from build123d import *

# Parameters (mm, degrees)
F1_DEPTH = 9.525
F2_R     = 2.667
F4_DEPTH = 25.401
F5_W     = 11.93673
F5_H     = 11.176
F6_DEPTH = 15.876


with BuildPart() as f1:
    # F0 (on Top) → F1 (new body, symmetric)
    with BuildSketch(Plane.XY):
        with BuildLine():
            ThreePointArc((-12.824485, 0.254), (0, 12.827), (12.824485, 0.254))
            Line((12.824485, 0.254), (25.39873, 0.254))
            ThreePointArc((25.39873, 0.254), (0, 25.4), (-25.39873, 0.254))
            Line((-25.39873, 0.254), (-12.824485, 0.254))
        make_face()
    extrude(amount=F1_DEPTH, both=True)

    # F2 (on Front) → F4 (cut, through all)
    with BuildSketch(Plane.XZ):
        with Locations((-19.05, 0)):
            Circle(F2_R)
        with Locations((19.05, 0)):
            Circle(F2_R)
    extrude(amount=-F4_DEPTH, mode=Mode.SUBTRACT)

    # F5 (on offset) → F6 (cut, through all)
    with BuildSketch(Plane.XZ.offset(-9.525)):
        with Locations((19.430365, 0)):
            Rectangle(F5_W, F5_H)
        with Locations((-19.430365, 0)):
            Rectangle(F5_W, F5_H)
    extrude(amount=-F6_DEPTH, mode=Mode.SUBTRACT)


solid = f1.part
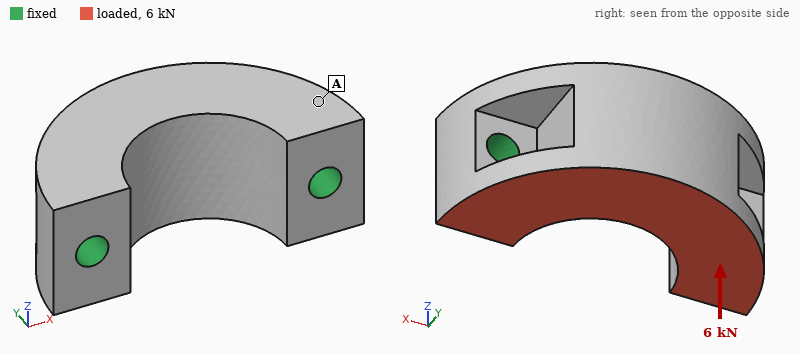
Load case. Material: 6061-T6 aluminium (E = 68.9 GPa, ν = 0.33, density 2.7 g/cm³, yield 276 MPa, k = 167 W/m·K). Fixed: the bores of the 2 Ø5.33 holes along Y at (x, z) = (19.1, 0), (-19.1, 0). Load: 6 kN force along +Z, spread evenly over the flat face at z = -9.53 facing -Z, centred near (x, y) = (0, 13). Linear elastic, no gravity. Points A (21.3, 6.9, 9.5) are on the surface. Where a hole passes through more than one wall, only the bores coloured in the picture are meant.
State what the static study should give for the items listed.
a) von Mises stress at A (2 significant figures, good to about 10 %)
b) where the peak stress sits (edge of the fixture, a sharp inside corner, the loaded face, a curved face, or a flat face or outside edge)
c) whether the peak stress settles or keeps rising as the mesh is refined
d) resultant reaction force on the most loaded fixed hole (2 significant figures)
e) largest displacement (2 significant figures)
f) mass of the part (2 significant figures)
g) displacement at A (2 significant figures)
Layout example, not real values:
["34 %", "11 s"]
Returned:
["31 MPa", "edge of the fixture", "keeps rising", "3.0 kN", "50 µm", "33 g", "8.2 µm"]
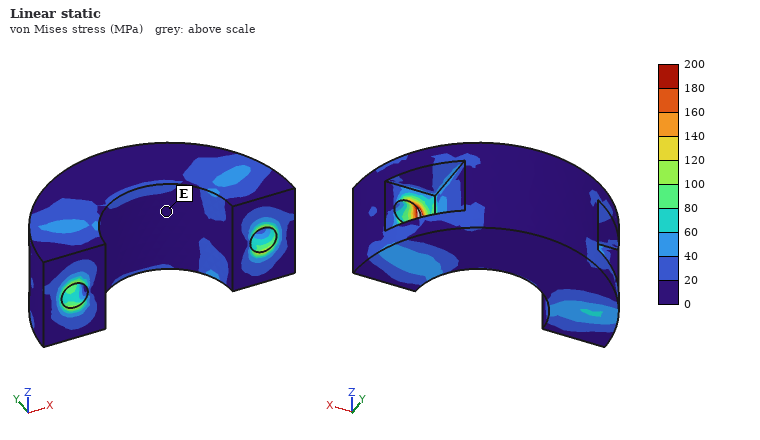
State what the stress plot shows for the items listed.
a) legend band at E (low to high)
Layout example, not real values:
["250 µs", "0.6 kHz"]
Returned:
["0 to 20 MPa"]
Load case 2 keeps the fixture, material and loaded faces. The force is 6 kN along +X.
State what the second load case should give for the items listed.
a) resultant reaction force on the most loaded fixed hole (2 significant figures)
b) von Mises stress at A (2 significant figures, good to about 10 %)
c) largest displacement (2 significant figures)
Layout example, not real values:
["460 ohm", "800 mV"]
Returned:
["3.3 kN", "14 MPa", "21 µm"]
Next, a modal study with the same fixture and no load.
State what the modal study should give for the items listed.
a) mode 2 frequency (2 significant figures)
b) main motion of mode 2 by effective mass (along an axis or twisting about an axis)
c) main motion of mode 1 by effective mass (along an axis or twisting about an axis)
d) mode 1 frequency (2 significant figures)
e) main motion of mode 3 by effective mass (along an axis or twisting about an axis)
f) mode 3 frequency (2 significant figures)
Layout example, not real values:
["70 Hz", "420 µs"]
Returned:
["25 kHz", "along X", "along Z", "11 kHz", "along Y", "27 kHz"]
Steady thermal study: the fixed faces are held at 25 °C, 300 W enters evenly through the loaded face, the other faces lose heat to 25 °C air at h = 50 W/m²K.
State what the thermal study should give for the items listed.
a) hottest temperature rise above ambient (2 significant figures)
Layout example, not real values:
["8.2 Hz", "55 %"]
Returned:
["75 K"]
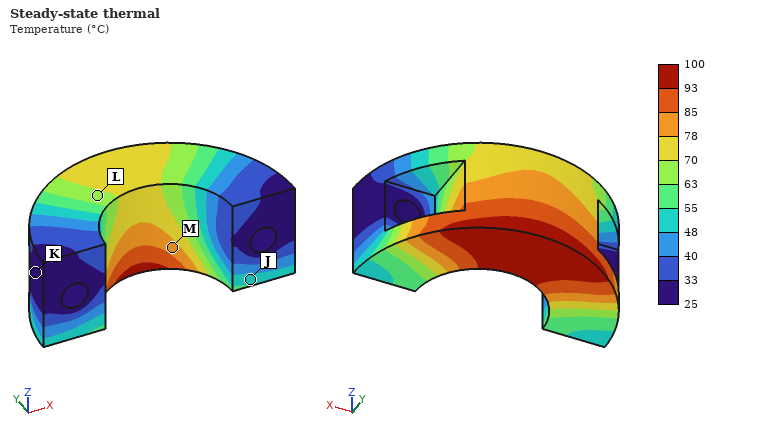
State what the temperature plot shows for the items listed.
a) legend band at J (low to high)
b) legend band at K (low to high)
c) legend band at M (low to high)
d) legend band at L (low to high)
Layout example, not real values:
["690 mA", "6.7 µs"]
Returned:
["48 to 55 °C", "25 to 33 °C", "78 to 85 °C", "63 to 70 °C"]
